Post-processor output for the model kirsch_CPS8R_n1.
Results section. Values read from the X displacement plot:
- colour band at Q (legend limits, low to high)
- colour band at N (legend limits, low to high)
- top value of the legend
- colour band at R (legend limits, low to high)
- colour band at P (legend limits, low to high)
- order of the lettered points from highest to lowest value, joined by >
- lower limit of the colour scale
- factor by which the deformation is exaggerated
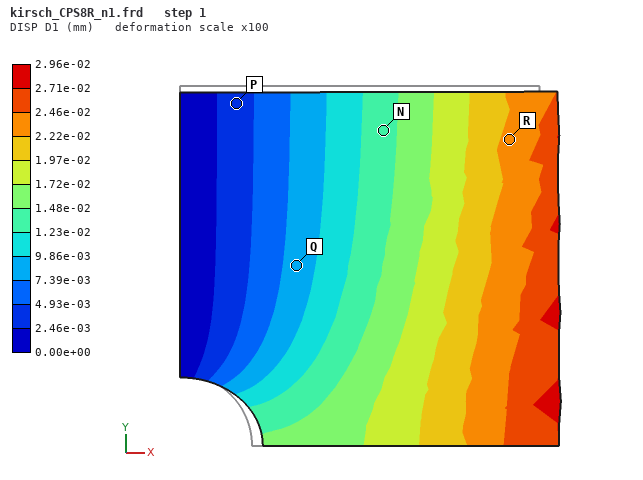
7.39e-03 to 9.86e-03 mm
1.23e-02 to 1.48e-02 mm
2.96e-02 mm
2.22e-02 to 2.46e-02 mm
2.46e-03 to 4.93e-03 mm
R > N > Q > P
0.00e+00 mm
100
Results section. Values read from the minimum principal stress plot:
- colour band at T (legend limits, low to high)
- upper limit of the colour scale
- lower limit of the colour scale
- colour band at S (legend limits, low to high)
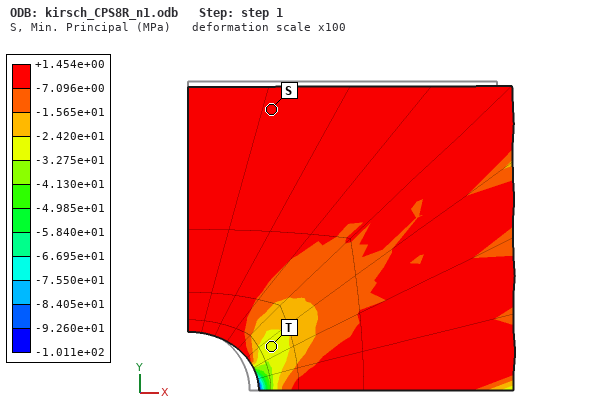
-3.275e+01 to -2.420e+01 MPa
+1.454e+00 MPa
-1.011e+02 MPa
-7.096e+00 to +1.454e+00 MPa
